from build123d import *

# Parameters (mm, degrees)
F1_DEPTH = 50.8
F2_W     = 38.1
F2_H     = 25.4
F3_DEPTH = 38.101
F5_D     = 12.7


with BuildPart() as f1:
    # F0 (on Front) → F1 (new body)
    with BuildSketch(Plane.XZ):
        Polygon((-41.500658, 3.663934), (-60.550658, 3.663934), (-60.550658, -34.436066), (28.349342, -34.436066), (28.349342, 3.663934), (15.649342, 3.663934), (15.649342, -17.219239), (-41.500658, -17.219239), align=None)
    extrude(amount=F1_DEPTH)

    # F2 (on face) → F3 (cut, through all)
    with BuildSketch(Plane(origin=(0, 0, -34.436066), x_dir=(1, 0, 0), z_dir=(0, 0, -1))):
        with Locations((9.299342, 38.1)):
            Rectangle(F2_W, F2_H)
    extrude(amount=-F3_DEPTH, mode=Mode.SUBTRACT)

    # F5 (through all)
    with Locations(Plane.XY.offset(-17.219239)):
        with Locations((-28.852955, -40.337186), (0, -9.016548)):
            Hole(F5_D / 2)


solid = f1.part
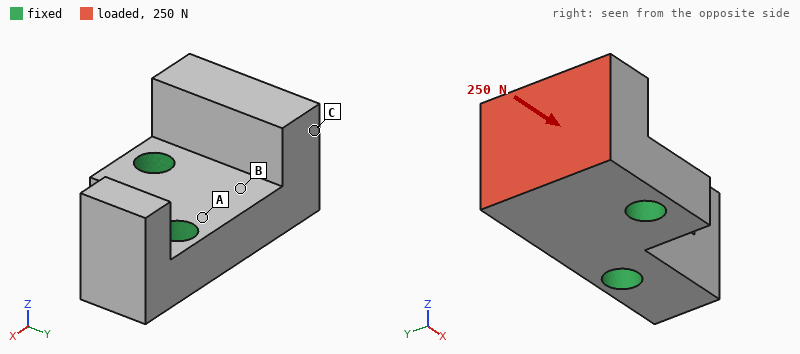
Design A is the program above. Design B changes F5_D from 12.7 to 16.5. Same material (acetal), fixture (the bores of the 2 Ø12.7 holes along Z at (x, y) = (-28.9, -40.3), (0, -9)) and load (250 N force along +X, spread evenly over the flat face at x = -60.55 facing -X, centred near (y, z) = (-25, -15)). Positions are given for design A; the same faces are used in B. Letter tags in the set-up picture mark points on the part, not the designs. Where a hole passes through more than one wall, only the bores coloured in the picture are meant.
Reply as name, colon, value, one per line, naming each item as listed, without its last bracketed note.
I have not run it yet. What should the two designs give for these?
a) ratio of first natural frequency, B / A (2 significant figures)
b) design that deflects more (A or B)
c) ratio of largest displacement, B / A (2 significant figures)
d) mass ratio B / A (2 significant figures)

ratio of first natural frequency, B / A: 1.1
design that deflects more: A
ratio of largest displacement, B / A: 0.88
mass ratio B / A: 0.96
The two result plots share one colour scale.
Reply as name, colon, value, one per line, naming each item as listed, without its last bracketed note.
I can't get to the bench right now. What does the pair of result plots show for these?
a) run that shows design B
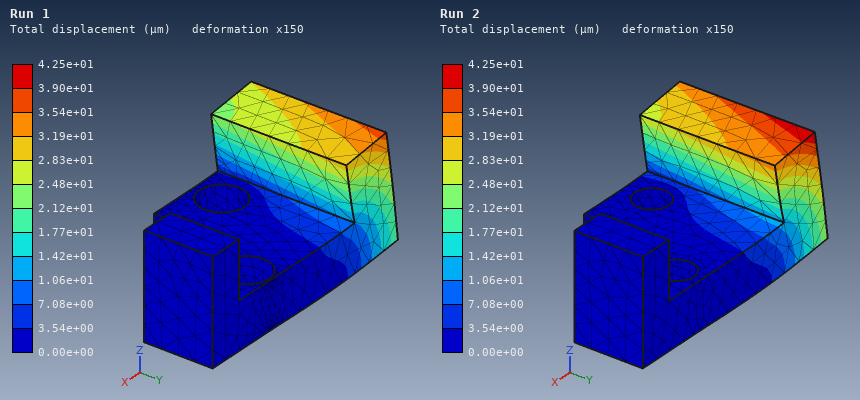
run that shows design B: Run 1
